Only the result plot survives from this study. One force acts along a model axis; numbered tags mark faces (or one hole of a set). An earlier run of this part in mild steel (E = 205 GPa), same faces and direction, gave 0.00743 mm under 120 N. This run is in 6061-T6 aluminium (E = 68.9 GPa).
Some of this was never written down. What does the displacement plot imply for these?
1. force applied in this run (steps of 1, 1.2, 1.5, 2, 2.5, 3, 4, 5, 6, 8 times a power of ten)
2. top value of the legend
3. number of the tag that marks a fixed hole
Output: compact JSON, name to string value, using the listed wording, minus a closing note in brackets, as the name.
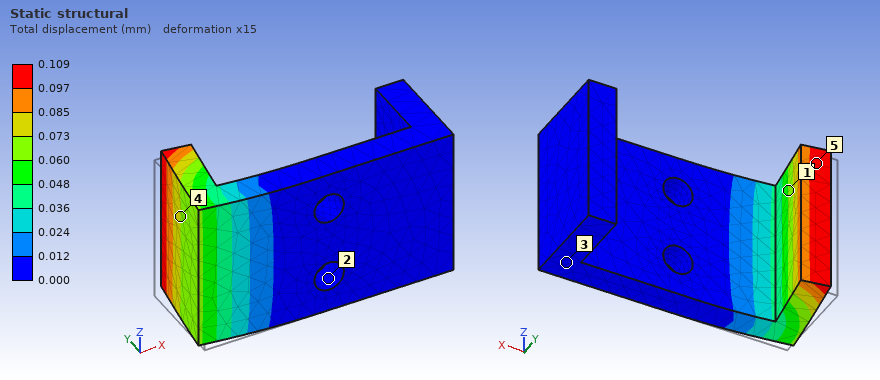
{"force applied in this run": "600 N", "top value of the legend": "0.109 mm", "number of the tag that marks a fixed hole": "2"}
